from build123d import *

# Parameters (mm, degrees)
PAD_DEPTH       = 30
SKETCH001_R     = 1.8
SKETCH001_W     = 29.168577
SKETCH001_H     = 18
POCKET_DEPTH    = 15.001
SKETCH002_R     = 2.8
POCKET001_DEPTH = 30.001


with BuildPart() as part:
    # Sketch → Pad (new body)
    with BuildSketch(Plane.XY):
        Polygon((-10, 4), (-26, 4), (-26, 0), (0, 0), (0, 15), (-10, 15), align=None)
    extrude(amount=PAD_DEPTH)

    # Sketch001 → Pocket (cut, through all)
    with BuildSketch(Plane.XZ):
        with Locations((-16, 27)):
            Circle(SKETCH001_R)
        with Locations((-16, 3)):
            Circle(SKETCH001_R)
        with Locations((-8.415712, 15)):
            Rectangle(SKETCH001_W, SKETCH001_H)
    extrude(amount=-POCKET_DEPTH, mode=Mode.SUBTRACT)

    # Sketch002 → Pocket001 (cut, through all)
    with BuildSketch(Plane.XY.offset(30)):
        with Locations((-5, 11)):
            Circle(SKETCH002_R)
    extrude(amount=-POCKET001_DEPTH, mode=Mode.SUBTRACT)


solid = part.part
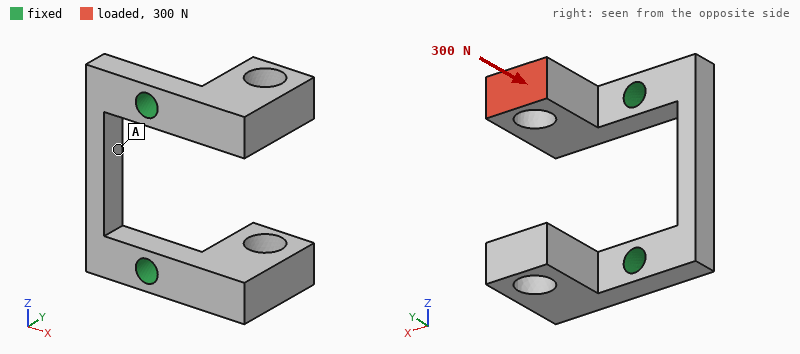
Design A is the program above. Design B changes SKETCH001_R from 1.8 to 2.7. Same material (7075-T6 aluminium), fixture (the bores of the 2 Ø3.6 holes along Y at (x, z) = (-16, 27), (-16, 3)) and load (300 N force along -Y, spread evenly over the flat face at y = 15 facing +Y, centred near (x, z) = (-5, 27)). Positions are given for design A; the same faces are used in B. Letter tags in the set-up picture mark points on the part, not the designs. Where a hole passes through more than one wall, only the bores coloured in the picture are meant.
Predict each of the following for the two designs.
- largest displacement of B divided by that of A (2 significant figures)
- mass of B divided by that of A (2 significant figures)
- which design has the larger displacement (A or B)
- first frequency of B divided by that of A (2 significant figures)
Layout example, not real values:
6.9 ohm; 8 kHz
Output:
0.75; 0.96; A; 1.1
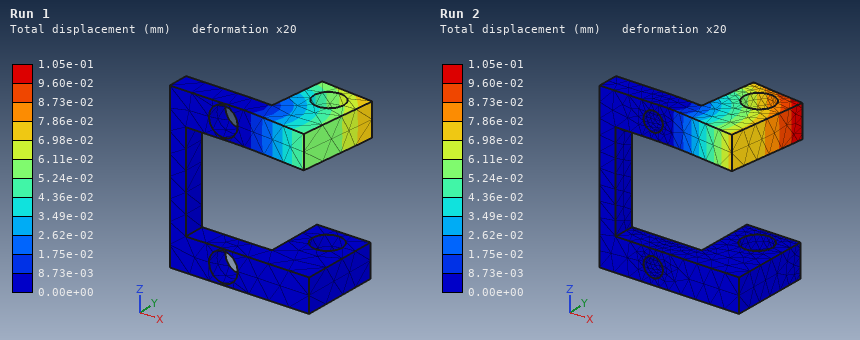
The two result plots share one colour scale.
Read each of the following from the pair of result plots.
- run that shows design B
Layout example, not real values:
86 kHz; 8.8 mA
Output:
Run 1
